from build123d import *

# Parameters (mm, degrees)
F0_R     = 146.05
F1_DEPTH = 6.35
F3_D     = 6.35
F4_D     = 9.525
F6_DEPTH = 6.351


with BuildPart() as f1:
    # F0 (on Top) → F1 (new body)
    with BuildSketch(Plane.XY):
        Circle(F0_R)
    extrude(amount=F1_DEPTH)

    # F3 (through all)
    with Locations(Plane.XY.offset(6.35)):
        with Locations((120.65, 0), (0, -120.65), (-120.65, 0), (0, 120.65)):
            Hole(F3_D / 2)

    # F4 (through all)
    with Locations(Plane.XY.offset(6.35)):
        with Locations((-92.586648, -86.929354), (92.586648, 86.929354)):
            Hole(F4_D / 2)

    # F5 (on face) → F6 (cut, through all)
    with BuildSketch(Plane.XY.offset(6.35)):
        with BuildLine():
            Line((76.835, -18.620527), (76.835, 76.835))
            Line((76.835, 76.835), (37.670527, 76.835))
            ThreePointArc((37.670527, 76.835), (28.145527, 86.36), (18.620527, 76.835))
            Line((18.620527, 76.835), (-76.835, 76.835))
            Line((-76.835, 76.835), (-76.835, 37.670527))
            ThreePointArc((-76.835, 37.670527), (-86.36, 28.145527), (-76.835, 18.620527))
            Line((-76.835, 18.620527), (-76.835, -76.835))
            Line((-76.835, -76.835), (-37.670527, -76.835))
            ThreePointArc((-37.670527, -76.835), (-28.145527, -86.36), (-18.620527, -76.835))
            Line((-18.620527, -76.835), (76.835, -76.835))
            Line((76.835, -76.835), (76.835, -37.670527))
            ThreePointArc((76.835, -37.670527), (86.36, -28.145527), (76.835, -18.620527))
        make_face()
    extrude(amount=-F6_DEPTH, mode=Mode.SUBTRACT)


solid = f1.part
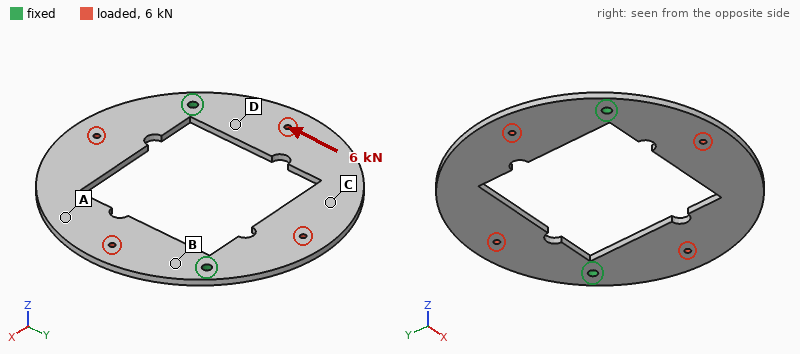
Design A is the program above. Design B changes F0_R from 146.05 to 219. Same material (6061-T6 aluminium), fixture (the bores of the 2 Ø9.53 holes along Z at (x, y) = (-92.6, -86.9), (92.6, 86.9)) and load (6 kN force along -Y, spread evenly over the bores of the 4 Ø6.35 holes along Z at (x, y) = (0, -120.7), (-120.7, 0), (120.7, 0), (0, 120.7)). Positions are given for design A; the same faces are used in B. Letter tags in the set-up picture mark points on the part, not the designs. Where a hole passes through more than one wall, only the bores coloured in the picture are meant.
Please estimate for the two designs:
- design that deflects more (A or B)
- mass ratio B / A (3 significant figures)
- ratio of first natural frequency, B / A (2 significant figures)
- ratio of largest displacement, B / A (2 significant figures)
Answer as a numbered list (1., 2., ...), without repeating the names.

1. A
2. 2.97
3. 0.53
4. 0.43
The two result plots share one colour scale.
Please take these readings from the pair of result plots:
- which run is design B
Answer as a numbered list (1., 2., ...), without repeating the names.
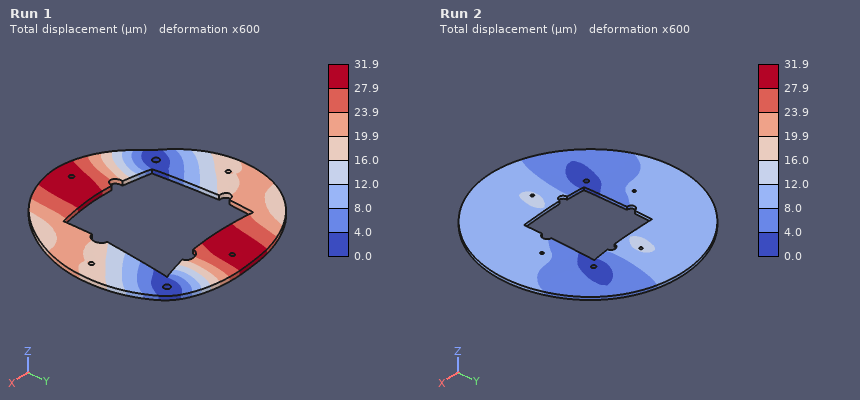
1. Run 2
